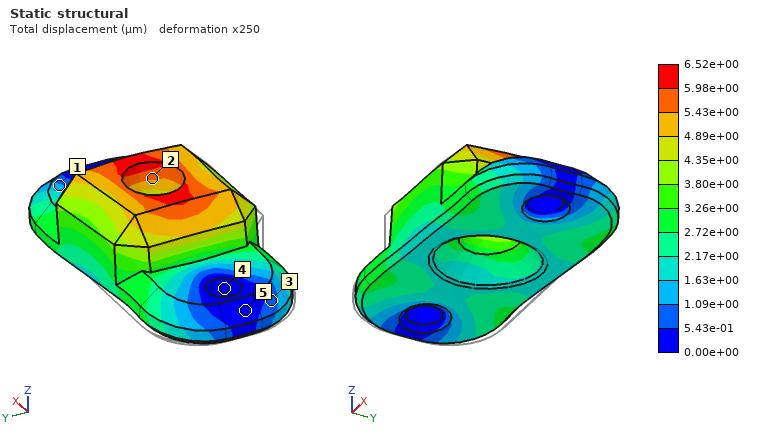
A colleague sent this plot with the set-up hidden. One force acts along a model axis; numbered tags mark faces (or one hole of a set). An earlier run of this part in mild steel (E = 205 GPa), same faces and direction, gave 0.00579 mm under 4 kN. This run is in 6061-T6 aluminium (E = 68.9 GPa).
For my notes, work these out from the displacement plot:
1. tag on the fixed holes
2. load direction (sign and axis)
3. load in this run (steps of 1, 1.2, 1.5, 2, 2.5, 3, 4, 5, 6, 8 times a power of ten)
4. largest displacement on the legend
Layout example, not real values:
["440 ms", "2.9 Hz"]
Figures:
["4", "+X", "1.5 kN", "6.52e+00 µm"]
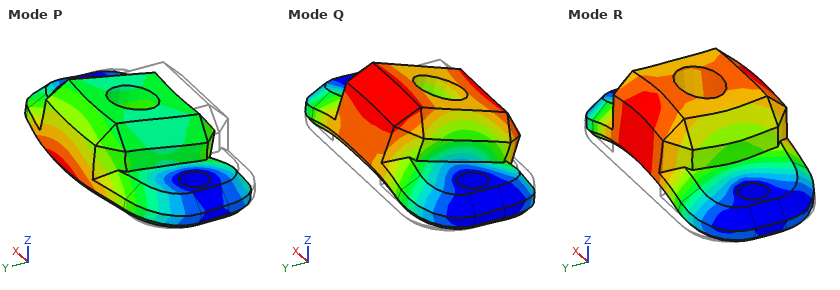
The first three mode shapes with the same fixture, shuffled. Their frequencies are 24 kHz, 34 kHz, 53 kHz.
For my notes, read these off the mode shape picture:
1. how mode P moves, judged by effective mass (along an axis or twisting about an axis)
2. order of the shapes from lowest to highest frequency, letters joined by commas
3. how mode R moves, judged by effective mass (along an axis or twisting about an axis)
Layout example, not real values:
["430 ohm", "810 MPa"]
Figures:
["along Y", "Q, R, P", "along Z"]
